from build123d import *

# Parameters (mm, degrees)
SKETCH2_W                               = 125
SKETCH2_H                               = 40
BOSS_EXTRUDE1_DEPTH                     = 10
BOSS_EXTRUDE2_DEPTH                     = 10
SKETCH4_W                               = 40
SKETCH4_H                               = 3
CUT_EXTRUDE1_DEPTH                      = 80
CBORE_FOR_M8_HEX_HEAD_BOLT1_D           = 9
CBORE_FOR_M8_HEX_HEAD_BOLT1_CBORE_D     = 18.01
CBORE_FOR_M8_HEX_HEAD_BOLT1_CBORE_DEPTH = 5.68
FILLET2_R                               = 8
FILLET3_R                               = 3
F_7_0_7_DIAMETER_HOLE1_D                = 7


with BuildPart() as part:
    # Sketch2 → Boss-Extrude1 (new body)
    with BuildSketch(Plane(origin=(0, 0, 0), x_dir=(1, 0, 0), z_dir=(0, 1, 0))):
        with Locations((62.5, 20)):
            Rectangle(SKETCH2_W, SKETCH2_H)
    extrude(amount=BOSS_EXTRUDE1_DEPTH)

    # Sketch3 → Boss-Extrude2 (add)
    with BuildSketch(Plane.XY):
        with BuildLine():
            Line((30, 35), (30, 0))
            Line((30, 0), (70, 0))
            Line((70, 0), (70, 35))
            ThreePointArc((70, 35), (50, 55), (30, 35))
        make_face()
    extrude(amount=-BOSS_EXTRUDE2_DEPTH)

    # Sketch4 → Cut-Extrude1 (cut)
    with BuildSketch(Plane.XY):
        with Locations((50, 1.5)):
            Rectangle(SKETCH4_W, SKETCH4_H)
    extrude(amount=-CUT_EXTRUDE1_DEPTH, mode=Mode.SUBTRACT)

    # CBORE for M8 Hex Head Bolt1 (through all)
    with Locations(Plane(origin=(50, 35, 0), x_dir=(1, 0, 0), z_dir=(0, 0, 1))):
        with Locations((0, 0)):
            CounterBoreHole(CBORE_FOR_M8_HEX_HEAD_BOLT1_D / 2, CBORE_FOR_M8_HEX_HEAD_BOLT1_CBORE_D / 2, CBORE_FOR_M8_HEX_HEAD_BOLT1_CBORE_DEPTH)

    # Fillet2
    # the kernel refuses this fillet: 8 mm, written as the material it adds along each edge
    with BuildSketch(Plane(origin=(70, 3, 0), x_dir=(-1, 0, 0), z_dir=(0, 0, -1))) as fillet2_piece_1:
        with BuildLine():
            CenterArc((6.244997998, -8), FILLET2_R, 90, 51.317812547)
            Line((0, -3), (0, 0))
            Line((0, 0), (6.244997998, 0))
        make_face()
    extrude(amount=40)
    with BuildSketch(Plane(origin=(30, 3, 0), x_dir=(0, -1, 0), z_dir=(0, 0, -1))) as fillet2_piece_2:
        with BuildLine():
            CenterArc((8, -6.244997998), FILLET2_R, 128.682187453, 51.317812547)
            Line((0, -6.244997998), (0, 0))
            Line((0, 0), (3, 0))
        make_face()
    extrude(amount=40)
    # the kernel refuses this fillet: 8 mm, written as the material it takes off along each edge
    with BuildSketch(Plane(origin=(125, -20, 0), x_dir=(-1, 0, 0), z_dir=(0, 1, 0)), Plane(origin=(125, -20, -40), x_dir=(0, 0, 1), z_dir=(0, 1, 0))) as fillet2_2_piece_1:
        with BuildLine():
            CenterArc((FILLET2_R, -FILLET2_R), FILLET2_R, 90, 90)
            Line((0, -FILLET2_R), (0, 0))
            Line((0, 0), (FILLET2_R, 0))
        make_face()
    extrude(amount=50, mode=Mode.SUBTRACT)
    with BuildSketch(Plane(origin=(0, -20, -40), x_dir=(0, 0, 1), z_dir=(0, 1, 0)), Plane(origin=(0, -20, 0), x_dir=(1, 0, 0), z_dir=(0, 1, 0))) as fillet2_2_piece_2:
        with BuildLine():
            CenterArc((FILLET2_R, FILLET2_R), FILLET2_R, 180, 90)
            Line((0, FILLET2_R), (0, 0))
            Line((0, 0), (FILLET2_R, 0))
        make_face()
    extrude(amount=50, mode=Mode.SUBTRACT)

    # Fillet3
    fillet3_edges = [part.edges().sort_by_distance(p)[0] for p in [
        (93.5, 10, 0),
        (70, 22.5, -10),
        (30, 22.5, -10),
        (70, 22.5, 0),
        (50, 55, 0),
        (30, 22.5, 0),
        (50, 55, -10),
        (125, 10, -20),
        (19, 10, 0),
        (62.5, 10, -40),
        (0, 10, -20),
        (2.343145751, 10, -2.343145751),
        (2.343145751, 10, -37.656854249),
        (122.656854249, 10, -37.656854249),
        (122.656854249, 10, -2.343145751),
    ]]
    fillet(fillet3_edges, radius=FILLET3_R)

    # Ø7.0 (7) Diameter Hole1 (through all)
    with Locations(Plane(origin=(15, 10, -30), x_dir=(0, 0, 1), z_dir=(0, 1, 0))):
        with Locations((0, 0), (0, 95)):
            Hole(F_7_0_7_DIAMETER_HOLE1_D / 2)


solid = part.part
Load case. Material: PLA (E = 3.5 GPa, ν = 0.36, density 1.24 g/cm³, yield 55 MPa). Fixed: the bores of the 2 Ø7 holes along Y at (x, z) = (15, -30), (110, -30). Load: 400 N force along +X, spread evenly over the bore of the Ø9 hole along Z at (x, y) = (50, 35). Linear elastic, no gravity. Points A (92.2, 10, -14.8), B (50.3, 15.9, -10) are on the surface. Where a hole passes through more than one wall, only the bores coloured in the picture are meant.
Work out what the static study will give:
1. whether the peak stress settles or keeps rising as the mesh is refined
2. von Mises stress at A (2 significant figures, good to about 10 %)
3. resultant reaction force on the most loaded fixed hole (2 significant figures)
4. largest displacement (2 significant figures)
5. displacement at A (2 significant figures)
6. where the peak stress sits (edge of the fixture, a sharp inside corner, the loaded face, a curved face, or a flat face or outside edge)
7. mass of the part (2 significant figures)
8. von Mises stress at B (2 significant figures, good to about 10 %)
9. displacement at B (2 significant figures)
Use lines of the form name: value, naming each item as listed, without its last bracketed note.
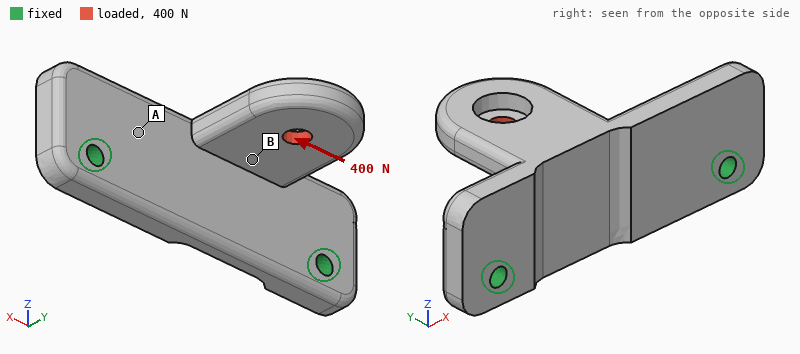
whether the peak stress settles or keeps rising as the mesh is refined: keeps rising
von Mises stress at A: 1.8 MPa
resultant reaction force on the most loaded fixed hole: 280 N
largest displacement: 0.47 mm
displacement at A: 0.099 mm
where the peak stress sits: a sharp inside corner
mass of the part: 72 g
von Mises stress at B: 4.4 MPa
displacement at B: 0.12 mm
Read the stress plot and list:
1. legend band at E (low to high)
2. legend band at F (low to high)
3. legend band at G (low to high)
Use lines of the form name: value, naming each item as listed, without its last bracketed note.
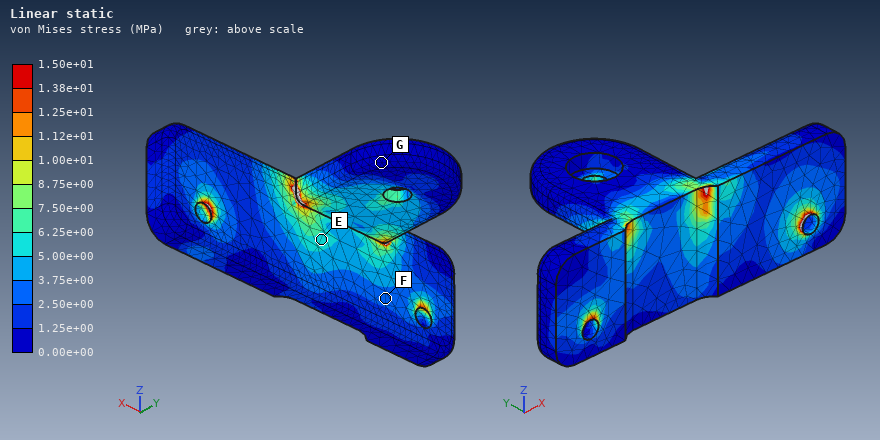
legend band at E: 5.00e+00 to 6.25e+00 MPa
legend band at F: 2.50e+00 to 3.75e+00 MPa
legend band at G: 0.00e+00 to 1.25e+00 MPa
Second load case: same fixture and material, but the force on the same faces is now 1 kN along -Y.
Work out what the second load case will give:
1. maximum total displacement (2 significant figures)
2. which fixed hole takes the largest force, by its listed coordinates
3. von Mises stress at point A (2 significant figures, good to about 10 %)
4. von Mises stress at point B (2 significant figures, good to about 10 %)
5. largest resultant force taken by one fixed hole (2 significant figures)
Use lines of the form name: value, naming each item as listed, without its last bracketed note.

maximum total displacement: 1.2 mm
which fixed hole takes the largest force, by its listed coordinates: (15, -30)
von Mises stress at point A: 7.7 MPa
von Mises stress at point B: 3.4 MPa
largest resultant force taken by one fixed hole: 670 N
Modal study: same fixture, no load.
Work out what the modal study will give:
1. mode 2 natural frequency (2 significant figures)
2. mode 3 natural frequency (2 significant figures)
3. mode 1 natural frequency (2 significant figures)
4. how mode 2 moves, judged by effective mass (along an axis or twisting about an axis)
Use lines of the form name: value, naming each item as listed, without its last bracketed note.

mode 2 natural frequency: 1100 Hz
mode 3 natural frequency: 1600 Hz
mode 1 natural frequency: 700 Hz
how mode 2 moves, judged by effective mass: along Y
